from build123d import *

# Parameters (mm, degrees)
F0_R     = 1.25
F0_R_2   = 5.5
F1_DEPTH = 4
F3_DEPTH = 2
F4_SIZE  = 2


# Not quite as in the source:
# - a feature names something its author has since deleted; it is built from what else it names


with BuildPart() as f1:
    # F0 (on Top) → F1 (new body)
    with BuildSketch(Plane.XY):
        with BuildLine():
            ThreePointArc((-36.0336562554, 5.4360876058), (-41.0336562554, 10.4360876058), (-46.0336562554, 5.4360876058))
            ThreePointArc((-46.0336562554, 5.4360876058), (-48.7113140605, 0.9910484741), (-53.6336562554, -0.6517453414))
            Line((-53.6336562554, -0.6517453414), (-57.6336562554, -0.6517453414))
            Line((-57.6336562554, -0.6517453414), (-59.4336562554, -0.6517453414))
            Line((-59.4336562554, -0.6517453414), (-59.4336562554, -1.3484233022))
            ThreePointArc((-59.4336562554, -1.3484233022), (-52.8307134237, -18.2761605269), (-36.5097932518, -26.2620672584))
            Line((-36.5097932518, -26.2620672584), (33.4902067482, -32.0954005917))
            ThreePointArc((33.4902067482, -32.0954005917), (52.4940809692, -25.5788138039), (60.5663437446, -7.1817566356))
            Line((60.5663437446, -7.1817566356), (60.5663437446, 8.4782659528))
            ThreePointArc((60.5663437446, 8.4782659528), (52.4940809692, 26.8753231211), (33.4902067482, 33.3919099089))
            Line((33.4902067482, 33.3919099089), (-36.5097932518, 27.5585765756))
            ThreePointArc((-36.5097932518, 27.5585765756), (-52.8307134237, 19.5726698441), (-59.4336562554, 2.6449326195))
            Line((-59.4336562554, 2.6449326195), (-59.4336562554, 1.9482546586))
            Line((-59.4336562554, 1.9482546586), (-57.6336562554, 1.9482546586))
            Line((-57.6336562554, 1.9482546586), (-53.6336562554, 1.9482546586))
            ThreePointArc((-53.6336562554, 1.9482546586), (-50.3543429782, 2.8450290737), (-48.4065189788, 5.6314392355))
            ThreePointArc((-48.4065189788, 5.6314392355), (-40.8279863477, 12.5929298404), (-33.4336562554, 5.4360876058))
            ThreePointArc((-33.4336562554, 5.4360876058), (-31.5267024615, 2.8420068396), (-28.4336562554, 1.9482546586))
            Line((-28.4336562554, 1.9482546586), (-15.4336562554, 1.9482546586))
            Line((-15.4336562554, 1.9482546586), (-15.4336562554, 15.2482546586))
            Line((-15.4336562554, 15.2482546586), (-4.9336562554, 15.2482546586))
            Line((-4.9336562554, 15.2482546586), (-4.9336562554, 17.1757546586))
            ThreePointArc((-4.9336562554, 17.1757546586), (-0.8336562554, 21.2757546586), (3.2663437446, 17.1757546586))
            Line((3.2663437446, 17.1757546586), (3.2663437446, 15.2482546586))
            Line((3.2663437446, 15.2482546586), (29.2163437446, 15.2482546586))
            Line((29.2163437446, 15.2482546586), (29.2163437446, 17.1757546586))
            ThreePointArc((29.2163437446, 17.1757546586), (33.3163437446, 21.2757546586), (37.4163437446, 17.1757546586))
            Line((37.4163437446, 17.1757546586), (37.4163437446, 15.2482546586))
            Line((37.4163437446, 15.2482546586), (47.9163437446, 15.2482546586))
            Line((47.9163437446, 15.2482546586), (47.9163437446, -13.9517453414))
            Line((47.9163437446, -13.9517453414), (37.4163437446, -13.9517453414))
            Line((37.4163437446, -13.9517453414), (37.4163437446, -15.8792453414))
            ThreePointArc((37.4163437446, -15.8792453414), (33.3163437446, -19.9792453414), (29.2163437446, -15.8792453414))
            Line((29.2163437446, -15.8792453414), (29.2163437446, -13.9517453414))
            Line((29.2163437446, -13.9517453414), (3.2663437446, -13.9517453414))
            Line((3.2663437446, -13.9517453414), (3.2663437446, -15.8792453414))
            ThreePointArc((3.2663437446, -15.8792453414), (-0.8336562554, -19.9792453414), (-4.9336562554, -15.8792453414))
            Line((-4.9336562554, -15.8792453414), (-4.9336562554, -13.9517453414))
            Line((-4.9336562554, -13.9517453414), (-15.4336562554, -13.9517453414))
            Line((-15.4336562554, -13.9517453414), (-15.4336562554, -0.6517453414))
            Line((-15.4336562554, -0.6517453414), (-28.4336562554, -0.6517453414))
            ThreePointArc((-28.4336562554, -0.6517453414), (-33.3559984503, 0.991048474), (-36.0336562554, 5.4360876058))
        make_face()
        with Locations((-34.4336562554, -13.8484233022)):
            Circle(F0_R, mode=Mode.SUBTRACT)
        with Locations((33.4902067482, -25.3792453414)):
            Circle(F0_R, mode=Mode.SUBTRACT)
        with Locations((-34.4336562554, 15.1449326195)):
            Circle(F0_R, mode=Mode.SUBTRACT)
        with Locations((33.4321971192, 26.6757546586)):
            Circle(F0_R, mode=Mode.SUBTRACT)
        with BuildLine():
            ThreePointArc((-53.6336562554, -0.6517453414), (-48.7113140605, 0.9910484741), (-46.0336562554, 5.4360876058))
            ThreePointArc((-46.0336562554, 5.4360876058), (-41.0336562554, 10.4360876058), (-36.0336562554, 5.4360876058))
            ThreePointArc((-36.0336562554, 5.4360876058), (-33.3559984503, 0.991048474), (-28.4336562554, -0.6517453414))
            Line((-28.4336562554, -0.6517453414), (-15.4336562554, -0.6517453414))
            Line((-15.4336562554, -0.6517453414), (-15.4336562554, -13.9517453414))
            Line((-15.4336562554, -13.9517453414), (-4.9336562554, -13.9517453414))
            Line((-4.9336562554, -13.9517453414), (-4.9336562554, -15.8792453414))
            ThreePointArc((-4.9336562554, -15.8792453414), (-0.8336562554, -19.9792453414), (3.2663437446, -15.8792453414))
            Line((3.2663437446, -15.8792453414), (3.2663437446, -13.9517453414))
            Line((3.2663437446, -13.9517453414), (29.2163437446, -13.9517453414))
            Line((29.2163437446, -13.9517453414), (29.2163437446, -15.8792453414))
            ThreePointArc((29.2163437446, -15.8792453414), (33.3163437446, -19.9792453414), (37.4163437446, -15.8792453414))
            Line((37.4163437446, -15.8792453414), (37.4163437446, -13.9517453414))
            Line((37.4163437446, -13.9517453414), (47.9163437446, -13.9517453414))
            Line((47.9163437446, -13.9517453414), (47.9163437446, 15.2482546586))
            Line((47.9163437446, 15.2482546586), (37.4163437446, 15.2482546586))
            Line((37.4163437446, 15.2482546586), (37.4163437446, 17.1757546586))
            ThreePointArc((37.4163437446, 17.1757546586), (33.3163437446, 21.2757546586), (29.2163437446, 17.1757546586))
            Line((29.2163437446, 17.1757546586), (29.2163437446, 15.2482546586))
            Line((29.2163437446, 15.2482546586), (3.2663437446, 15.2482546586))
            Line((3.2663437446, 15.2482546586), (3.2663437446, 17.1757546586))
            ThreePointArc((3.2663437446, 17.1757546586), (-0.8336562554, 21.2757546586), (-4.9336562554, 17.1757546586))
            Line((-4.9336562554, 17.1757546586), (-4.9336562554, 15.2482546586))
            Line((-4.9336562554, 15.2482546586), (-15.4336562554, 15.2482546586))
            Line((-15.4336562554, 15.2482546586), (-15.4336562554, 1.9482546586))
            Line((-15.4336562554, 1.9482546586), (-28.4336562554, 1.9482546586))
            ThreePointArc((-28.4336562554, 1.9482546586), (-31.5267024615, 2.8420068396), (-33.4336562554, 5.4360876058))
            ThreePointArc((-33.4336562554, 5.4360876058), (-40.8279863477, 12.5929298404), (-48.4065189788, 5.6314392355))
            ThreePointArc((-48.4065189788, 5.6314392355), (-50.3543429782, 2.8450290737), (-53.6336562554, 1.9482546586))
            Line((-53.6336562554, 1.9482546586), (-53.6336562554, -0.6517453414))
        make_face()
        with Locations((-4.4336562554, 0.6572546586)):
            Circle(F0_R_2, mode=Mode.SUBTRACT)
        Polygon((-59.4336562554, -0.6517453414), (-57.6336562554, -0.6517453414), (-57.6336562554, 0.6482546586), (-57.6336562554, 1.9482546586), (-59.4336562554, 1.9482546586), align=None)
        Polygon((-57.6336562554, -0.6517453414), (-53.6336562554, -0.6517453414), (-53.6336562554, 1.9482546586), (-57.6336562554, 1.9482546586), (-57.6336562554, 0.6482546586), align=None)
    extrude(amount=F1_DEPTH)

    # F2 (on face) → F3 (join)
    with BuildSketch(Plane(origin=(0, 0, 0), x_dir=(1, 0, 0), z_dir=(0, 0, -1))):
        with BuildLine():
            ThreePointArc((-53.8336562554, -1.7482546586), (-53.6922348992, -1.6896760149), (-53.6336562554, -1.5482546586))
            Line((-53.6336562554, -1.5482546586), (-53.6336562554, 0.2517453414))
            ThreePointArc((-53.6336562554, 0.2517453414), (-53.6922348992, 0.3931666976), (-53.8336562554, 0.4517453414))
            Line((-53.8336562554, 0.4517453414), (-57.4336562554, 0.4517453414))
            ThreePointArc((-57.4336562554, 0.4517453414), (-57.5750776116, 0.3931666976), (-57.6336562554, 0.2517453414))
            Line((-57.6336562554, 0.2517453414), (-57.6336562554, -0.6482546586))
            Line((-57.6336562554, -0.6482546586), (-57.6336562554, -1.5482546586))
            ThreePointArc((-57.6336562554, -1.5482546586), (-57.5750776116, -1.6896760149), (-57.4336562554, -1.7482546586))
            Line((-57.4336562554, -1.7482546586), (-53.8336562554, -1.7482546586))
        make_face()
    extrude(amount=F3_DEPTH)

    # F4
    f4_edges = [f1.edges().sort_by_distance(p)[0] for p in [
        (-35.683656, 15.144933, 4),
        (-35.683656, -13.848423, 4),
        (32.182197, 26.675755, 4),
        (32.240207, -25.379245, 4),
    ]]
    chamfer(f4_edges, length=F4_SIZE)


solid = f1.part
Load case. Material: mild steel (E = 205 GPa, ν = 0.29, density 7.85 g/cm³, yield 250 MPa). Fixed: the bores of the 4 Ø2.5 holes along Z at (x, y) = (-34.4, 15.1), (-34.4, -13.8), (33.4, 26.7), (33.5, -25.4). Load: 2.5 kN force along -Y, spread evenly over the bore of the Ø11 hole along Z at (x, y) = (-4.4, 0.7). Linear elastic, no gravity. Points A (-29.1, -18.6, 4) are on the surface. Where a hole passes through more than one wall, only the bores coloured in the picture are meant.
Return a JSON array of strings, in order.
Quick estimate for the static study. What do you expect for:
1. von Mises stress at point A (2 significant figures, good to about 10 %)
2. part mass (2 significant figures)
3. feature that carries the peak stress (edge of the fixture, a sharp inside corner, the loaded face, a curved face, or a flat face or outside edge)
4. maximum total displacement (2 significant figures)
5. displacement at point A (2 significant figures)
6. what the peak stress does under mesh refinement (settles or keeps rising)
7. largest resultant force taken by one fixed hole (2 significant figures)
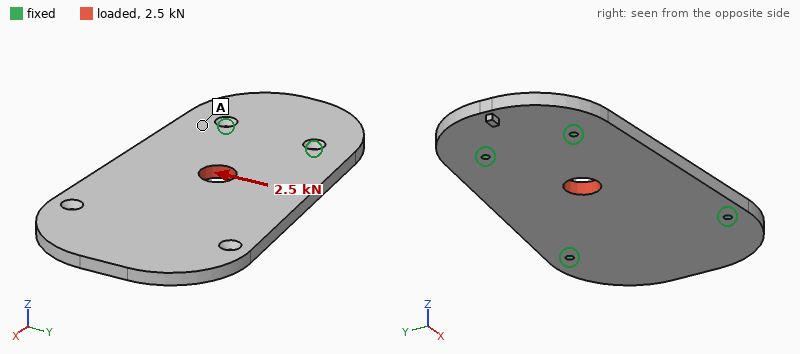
["6.0 MPa", "200 g", "edge of the fixture", "3.9 µm", "1.3 µm", "keeps rising", "740 N"]
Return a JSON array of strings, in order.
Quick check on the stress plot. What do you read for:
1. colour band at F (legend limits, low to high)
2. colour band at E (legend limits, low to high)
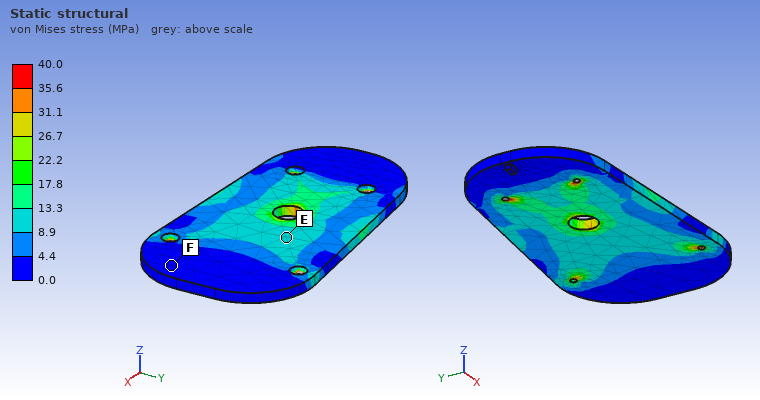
["0.0 to 4.4 MPa", "8.9 to 13.3 MPa"]
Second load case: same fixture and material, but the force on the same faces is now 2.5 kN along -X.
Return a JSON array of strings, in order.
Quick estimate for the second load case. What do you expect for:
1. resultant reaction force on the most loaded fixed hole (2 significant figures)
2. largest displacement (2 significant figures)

["700 N", "3.4 µm"]
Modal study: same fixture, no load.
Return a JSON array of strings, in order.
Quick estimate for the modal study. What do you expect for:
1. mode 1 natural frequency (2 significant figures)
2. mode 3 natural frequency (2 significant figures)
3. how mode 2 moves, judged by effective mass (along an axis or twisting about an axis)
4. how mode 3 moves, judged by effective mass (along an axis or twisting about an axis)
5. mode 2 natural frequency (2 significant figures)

["2600 Hz", "4500 Hz", "along Z", "twisting about X", "3300 Hz"]
